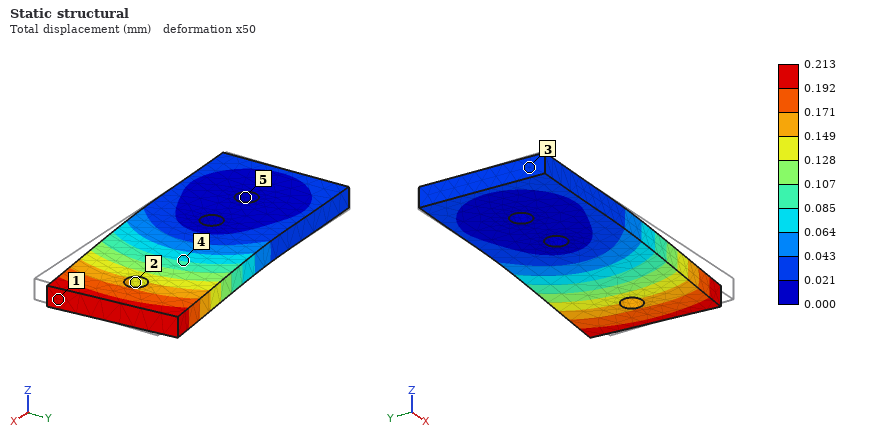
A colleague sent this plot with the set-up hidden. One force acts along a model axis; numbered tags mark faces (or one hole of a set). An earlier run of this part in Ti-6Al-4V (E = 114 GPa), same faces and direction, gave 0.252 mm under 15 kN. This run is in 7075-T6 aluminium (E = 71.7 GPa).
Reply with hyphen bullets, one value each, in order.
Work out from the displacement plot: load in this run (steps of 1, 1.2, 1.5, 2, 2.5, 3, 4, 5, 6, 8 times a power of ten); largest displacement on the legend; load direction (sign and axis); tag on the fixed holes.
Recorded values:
- 8 kN
- 0.213 mm
- +Y
- 5
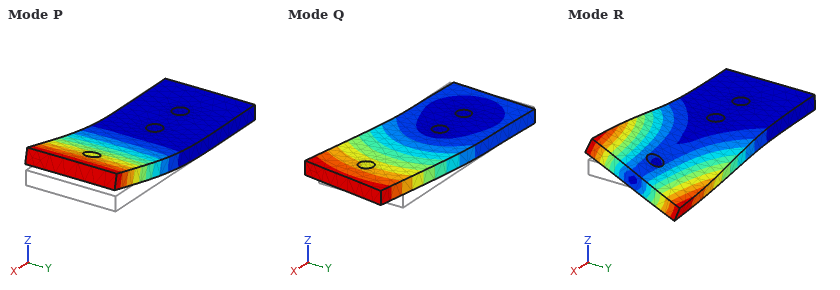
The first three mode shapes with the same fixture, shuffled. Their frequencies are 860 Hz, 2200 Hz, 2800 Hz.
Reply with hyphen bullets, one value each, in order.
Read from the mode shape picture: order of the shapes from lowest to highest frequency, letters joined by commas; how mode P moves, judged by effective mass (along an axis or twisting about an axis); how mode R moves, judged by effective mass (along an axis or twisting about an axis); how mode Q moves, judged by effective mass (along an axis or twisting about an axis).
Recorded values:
- P, R, Q
- along Z
- twisting about X
- along Y
